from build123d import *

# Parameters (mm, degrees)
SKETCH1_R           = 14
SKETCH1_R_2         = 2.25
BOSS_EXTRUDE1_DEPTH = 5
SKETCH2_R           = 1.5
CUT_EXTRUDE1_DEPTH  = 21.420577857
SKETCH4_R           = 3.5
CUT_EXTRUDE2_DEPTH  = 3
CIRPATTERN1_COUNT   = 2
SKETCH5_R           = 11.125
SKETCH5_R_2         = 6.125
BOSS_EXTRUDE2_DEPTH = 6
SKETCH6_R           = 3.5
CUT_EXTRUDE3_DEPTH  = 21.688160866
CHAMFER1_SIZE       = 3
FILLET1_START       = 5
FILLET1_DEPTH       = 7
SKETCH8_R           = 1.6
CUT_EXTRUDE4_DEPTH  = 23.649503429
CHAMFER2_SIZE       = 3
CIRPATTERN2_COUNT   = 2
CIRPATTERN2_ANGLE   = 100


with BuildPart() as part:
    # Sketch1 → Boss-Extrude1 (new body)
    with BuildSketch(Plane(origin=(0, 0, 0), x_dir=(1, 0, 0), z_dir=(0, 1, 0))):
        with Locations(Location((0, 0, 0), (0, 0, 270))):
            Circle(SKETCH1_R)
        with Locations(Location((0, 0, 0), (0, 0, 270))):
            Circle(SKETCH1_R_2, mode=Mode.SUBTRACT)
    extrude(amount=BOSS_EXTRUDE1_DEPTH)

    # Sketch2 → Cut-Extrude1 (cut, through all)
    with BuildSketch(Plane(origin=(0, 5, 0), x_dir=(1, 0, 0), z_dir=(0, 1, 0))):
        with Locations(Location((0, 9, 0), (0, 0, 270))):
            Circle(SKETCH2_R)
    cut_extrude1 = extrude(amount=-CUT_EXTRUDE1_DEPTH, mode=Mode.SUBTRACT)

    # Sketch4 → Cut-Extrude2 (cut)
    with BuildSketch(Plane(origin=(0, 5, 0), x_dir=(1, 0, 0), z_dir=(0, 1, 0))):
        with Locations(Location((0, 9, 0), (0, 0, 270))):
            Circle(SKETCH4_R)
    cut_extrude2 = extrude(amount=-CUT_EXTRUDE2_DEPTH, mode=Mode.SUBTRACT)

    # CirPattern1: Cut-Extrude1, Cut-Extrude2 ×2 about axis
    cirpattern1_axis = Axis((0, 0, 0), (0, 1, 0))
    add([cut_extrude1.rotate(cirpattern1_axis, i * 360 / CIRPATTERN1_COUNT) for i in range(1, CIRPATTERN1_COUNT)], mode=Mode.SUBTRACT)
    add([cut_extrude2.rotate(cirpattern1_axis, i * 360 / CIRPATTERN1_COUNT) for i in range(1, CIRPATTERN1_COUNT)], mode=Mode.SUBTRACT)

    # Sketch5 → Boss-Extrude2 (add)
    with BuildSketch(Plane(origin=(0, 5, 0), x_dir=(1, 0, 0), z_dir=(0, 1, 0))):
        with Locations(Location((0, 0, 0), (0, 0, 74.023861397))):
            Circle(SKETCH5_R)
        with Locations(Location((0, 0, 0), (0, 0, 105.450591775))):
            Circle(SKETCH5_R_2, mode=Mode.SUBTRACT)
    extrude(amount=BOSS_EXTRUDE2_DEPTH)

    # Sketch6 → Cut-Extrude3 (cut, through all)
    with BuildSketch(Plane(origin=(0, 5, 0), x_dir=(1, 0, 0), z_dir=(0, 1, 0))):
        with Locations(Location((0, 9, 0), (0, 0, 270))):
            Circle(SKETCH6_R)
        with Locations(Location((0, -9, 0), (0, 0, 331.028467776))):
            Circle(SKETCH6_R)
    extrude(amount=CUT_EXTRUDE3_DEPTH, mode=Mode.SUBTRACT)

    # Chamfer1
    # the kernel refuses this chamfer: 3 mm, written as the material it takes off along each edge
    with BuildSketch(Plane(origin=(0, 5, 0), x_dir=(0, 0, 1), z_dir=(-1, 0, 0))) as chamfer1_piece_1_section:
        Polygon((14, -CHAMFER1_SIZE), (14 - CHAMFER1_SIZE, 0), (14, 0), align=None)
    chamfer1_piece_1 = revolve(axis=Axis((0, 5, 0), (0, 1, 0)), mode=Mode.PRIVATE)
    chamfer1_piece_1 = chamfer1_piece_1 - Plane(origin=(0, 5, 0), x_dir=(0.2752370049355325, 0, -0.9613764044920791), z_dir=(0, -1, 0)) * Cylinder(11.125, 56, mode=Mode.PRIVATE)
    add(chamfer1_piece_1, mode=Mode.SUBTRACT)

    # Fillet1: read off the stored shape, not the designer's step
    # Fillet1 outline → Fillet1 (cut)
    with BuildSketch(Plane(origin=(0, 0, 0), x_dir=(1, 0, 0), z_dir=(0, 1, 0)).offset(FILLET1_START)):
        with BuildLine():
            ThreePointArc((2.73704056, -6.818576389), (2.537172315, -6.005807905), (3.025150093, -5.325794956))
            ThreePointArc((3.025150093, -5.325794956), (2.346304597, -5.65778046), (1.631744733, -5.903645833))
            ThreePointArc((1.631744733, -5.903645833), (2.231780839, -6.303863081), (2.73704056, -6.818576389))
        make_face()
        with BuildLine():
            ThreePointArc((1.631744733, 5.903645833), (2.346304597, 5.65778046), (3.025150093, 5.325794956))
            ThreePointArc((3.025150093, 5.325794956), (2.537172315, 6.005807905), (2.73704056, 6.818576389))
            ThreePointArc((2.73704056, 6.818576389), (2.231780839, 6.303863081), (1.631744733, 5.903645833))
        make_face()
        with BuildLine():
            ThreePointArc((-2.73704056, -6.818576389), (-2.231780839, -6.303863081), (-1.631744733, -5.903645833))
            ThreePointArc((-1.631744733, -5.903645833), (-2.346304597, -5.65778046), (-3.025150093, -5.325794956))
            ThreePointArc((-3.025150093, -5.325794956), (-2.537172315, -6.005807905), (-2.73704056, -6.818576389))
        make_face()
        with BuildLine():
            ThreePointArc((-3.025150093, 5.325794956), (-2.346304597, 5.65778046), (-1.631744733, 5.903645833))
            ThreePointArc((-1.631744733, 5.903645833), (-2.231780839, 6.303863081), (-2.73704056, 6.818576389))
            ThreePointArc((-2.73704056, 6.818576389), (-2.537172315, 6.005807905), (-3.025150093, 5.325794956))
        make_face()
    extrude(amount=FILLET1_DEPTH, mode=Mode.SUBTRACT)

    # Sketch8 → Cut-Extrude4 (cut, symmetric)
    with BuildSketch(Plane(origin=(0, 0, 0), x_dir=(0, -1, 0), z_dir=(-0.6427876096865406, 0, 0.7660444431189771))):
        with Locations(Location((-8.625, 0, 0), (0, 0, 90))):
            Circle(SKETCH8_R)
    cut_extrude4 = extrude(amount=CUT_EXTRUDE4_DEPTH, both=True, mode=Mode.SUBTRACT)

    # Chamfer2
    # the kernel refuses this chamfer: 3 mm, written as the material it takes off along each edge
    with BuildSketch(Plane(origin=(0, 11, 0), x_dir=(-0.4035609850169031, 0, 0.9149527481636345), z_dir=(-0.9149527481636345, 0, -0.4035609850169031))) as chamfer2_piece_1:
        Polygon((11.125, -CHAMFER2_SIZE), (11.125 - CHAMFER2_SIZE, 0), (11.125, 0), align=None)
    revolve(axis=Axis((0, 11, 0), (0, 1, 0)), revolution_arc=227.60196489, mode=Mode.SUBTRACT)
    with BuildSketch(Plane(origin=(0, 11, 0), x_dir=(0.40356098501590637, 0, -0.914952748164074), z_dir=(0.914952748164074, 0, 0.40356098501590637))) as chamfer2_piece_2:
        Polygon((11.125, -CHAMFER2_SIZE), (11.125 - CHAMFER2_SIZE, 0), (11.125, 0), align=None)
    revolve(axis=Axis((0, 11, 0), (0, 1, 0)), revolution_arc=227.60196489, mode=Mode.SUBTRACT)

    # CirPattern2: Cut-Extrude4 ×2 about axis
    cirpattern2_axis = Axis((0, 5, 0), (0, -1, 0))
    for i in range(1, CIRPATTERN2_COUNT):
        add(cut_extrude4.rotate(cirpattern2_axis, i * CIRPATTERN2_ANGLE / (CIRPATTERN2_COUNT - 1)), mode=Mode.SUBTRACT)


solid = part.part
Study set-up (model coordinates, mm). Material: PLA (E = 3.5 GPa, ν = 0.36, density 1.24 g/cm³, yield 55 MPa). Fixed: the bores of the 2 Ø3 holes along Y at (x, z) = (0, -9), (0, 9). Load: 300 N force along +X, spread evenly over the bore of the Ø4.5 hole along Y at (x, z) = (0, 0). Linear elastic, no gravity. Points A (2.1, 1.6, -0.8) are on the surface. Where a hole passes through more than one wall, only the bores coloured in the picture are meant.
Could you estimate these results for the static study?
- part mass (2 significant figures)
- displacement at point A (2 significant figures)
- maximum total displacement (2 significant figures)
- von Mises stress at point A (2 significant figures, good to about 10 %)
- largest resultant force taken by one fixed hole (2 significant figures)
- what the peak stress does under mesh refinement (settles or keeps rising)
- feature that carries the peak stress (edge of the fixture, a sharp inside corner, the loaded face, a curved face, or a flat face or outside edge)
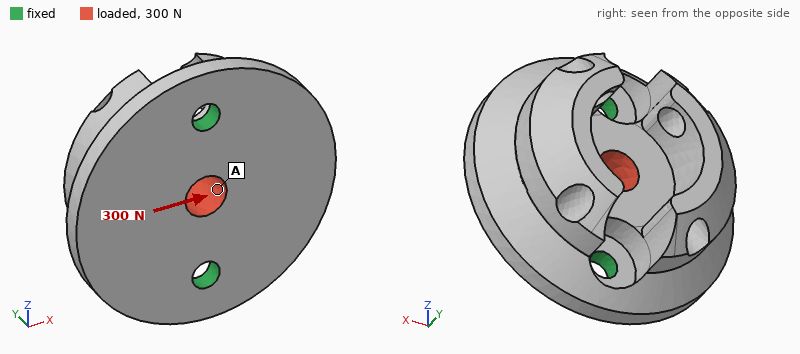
4.0 g
0.028 mm
0.11 mm
4.2 MPa
150 N
keeps rising
edge of the fixture
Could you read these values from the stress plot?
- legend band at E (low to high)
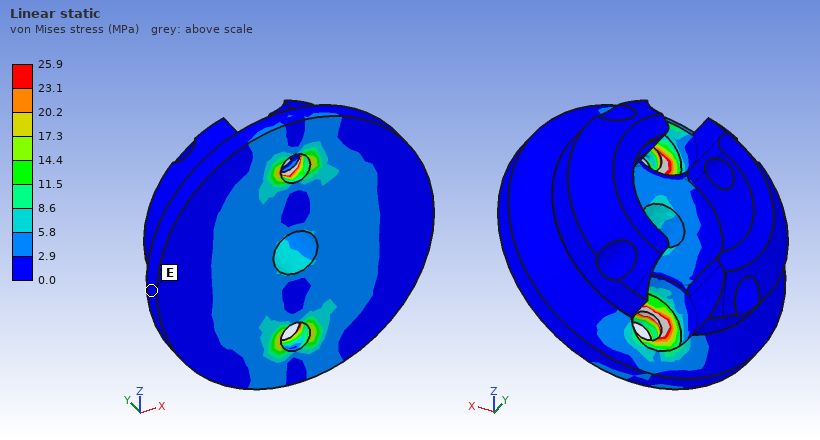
0.0 to 2.9 MPa
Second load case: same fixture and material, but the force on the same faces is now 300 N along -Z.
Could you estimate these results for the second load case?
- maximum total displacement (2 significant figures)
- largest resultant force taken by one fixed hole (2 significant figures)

18 µm
150 N
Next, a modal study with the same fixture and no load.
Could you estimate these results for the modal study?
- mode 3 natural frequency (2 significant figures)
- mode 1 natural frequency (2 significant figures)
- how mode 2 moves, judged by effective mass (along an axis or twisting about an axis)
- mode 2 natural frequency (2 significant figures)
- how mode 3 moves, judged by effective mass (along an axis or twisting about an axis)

10 kHz
2500 Hz
along Y
5300 Hz
along Z
